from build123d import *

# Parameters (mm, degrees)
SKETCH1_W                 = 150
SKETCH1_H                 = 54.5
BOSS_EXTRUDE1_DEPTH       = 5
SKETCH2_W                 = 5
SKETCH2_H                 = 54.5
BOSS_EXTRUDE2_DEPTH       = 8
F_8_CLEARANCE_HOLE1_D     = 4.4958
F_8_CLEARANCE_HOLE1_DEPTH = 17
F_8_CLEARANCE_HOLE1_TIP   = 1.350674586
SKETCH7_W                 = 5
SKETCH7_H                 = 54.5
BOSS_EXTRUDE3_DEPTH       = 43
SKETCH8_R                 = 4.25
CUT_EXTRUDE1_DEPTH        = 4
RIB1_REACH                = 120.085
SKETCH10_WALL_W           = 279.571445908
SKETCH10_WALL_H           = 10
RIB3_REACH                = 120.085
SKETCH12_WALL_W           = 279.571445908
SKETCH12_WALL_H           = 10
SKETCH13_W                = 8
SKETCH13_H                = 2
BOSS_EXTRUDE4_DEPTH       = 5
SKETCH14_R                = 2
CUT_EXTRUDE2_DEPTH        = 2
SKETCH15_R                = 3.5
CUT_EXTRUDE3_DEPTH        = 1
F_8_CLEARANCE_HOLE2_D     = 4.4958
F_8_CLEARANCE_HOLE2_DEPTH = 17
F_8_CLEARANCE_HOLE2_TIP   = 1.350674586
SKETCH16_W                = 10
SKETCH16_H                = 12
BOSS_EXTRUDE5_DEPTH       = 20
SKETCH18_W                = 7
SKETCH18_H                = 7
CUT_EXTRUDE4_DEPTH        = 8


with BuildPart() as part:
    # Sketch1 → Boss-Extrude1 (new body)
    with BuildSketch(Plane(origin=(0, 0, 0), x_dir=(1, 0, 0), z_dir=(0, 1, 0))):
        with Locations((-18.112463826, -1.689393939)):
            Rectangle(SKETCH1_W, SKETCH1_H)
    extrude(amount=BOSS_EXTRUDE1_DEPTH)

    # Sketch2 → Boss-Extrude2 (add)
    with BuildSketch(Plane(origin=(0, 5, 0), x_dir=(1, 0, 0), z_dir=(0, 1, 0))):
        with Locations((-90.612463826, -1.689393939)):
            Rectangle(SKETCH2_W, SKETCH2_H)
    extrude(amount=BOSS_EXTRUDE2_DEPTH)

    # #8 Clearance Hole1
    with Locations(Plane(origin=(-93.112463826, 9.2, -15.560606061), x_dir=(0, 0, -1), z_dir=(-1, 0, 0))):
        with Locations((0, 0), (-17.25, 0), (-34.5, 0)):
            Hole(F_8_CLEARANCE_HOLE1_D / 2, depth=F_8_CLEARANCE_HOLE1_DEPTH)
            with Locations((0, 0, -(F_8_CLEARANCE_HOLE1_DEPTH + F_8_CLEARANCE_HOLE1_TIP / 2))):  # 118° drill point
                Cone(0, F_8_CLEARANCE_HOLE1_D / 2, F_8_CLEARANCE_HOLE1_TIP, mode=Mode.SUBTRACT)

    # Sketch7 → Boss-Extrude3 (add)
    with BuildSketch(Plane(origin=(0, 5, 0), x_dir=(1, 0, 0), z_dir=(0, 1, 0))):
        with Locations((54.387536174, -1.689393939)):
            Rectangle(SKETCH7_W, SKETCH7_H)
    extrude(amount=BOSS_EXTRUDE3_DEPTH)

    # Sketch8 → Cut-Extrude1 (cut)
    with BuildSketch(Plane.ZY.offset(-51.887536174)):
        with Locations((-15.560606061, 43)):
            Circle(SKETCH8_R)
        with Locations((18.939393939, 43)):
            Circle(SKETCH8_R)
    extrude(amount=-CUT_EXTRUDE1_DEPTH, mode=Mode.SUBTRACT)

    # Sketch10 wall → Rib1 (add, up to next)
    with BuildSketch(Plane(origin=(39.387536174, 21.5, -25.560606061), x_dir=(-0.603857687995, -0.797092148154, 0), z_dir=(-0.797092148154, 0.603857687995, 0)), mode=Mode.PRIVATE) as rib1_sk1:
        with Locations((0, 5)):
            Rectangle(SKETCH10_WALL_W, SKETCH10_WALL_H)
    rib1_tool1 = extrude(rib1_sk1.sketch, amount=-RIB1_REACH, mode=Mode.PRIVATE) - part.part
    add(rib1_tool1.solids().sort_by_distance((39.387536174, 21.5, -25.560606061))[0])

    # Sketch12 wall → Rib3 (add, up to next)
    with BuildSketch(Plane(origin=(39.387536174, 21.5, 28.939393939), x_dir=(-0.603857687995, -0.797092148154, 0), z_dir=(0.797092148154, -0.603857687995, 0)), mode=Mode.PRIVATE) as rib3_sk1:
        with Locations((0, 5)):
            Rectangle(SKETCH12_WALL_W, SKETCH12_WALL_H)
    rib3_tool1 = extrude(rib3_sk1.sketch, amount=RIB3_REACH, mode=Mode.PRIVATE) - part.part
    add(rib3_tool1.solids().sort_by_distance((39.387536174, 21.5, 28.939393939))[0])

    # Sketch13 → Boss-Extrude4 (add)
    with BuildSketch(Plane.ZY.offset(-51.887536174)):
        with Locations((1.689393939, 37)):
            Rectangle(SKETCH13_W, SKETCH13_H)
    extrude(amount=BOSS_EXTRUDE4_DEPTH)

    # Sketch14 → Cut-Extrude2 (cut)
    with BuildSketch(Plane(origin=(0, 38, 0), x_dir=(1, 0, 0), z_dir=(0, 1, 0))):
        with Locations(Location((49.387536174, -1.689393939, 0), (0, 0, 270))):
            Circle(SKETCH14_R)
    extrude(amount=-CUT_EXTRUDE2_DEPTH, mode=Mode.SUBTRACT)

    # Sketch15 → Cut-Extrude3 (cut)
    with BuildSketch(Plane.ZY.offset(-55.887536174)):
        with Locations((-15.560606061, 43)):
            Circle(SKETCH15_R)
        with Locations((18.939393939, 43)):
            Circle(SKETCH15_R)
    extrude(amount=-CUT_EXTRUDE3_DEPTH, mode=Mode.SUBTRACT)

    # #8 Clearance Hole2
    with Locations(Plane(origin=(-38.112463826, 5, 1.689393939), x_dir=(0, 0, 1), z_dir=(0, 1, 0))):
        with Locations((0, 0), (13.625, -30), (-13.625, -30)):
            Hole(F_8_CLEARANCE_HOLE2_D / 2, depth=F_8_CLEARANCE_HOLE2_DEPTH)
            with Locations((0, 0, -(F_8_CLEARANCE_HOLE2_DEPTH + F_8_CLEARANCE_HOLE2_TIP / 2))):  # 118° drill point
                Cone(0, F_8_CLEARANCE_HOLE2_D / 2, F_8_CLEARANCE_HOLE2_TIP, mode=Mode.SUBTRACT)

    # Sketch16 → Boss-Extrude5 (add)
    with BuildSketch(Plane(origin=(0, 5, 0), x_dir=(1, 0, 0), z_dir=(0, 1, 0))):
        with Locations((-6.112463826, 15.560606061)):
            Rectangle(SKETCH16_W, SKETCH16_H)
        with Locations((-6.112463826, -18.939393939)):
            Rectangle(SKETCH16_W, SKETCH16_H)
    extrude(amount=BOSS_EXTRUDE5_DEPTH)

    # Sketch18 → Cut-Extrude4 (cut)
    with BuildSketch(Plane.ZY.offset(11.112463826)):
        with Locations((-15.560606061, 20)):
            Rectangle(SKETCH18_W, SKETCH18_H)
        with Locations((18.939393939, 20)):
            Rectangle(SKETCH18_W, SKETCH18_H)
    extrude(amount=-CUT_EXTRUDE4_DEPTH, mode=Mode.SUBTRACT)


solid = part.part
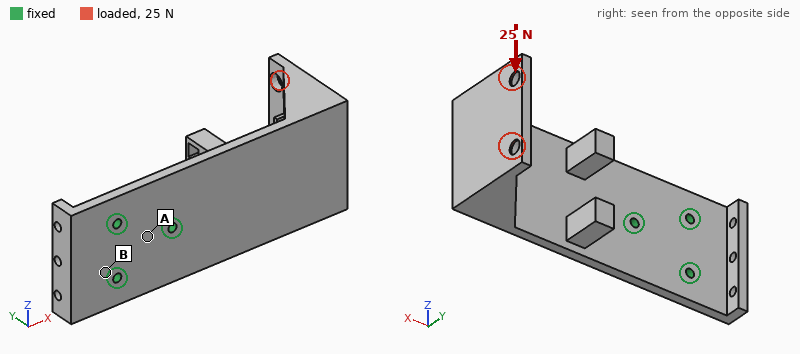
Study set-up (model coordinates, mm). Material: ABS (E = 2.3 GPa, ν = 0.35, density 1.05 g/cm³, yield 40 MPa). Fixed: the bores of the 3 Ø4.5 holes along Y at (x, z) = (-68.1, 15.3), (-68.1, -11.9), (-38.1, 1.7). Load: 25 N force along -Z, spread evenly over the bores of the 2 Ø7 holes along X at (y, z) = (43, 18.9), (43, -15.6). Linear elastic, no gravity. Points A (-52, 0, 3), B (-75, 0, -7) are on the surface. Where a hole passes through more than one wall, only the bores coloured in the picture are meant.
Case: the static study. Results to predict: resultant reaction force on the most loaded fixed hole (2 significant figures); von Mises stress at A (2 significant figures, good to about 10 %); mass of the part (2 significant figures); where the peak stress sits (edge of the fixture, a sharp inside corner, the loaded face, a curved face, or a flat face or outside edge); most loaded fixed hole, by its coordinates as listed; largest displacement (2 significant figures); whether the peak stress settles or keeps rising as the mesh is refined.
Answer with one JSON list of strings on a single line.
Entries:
["61 N", "0.93 MPa", "69 g", "edge of the fixture", "(-38.1, 1.7)", "1.8 mm", "keeps rising"]
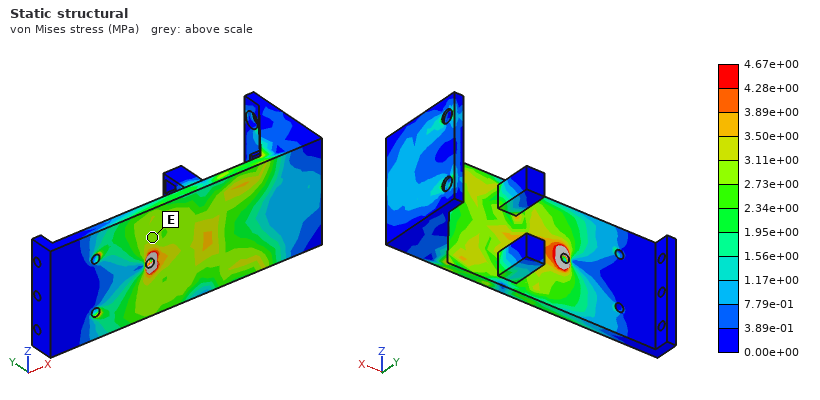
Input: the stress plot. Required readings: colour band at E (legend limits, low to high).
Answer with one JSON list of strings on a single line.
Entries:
["2.73e+00 to 3.11e+00 MPa"]
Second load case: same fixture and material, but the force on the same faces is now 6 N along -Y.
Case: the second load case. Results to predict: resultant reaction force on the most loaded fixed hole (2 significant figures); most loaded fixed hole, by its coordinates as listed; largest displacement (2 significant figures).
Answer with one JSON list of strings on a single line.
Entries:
["18 N", "(-38.1, 1.7)", "1.5 mm"]
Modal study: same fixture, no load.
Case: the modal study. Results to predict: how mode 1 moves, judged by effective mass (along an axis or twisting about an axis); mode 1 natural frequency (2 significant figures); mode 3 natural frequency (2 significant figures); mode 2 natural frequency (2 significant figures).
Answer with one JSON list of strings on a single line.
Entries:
["along Y", "68 Hz", "410 Hz", "190 Hz"]
